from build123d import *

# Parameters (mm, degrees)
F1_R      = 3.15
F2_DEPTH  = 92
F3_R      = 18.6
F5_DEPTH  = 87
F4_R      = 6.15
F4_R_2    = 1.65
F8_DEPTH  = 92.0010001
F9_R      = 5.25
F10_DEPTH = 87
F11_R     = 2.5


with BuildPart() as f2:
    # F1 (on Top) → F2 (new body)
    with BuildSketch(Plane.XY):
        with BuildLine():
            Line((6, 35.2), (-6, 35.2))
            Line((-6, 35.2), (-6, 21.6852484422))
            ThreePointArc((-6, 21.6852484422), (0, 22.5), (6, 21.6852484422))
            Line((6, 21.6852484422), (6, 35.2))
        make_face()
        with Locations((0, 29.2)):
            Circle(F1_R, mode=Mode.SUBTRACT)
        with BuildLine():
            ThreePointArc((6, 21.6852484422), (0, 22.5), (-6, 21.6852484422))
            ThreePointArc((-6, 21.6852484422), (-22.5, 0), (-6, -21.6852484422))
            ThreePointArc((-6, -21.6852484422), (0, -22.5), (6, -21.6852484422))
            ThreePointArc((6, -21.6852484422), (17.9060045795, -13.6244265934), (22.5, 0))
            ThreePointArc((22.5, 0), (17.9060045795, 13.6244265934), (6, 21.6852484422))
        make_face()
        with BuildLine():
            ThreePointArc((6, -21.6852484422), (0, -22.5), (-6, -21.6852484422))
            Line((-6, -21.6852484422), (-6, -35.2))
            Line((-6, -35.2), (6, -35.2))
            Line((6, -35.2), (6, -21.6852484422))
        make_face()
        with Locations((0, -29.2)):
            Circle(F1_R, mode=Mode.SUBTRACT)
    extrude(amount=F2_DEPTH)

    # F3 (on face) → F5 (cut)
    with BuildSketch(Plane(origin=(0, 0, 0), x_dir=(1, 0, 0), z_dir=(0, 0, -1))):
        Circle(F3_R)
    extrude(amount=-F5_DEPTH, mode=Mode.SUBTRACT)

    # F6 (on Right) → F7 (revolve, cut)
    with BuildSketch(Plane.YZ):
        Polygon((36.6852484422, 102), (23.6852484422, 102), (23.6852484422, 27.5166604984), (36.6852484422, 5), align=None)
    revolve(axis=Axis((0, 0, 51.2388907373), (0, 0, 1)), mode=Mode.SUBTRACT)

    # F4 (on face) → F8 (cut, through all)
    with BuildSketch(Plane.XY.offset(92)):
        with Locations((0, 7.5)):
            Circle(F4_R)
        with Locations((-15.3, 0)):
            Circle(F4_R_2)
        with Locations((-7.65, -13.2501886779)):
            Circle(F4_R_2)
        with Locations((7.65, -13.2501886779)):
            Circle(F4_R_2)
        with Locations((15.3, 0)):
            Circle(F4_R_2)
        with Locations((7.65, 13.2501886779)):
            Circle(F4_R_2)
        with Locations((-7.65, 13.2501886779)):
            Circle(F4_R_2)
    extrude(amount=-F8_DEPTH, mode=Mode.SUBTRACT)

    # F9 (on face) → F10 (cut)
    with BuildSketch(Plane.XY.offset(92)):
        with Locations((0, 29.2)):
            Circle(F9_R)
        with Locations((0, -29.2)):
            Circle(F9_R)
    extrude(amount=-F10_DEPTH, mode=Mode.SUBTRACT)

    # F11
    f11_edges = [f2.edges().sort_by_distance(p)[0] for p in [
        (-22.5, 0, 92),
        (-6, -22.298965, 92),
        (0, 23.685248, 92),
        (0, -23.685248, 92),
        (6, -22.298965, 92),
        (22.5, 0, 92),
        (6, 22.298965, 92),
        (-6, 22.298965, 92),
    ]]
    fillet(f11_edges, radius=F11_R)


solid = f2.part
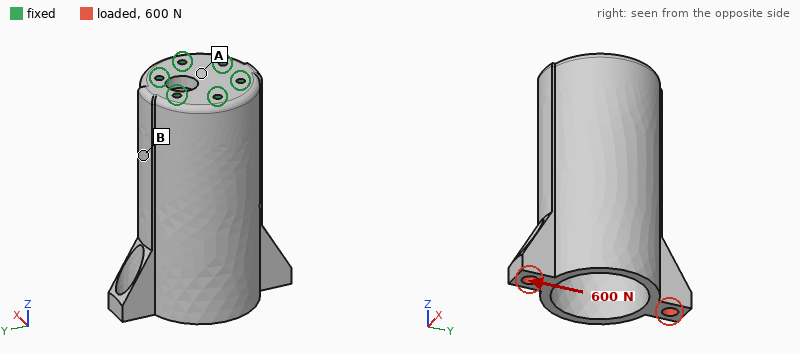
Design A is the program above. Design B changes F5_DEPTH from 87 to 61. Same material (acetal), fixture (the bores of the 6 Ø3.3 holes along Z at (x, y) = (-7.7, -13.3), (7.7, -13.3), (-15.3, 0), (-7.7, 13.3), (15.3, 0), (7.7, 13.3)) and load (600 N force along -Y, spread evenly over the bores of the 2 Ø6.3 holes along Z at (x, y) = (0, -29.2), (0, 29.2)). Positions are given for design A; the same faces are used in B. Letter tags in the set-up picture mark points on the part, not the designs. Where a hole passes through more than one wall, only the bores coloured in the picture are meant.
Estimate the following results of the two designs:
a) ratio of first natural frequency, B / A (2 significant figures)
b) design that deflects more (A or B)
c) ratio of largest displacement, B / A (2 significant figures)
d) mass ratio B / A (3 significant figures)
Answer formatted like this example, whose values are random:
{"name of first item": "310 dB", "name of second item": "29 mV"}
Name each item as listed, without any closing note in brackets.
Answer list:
{"ratio of first natural frequency, B / A": "2.2", "design that deflects more": "A", "ratio of largest displacement, B / A": "0.36", "mass ratio B / A": "1.43"}
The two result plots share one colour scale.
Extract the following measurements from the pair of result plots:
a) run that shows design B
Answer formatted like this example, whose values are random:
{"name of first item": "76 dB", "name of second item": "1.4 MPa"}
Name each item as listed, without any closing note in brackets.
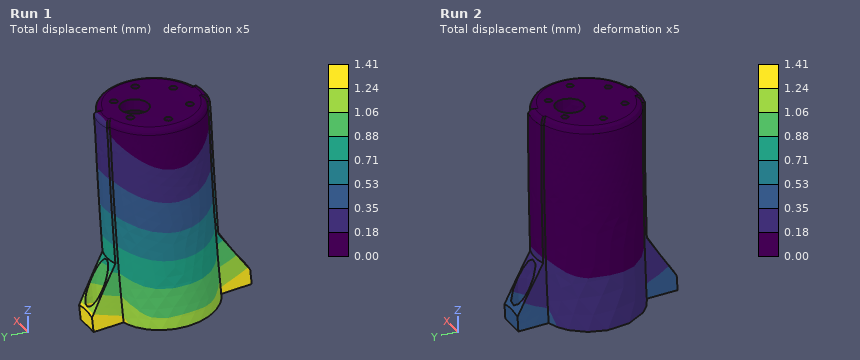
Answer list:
{"run that shows design B": "Run 2"}
